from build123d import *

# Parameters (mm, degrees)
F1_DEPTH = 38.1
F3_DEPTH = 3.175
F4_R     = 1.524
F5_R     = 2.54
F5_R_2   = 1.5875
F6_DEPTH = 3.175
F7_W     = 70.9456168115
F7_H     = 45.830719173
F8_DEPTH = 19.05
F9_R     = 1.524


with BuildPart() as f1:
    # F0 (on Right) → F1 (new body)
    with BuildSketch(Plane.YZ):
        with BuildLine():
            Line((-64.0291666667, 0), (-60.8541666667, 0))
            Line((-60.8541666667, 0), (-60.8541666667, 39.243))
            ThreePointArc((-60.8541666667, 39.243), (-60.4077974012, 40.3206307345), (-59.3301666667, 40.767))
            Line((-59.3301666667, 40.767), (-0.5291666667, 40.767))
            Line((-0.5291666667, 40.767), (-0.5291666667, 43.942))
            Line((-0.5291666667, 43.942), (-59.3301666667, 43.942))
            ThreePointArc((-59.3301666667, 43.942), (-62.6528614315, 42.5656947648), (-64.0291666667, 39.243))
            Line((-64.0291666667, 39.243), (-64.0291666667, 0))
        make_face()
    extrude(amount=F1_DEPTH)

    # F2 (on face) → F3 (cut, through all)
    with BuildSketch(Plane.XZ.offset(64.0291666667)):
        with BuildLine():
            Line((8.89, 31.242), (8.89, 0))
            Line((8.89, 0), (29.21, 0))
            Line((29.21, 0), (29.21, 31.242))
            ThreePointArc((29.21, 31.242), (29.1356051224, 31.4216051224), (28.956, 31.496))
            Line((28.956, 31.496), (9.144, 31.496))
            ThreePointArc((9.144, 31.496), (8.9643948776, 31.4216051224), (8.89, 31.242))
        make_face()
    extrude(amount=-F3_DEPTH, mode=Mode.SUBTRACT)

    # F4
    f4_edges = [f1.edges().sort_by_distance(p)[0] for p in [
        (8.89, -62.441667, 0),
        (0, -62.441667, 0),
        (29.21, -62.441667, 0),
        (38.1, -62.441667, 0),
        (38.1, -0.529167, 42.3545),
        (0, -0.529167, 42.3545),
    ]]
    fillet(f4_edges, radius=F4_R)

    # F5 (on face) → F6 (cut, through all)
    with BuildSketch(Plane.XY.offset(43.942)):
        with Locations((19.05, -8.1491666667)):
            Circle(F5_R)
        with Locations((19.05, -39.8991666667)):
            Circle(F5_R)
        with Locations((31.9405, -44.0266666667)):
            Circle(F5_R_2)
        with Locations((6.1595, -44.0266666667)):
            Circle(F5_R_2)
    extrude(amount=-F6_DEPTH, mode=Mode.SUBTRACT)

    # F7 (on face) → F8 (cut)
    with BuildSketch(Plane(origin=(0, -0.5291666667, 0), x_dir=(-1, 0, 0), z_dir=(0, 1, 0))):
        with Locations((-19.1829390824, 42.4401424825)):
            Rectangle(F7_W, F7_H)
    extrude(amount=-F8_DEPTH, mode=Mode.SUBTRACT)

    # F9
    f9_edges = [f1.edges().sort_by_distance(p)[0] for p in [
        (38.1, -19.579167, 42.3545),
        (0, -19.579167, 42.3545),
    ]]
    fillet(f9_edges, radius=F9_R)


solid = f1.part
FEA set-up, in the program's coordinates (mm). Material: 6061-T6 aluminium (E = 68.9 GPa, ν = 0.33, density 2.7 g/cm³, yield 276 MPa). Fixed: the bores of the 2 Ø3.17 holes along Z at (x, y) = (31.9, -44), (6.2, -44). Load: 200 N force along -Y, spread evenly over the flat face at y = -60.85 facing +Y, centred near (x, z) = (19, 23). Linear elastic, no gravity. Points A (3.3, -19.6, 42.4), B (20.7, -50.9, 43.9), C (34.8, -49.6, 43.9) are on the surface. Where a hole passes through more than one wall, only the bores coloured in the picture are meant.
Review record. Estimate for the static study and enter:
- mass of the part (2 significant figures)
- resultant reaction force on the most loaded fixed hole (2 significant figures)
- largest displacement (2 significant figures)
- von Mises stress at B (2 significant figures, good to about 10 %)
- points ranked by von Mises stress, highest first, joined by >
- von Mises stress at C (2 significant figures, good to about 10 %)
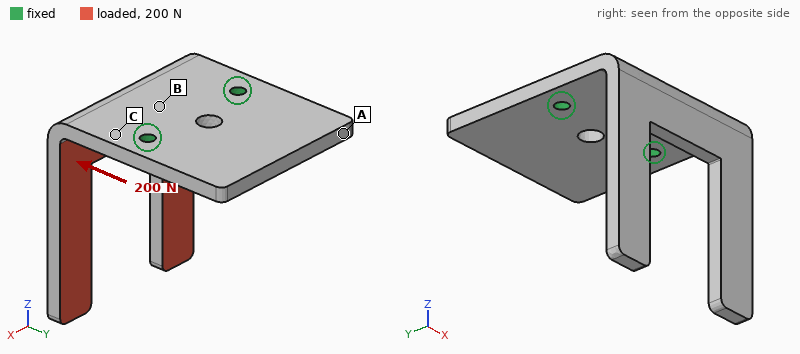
22 g
100 N
0.80 mm
47 MPa
C > B > A
64 MPa
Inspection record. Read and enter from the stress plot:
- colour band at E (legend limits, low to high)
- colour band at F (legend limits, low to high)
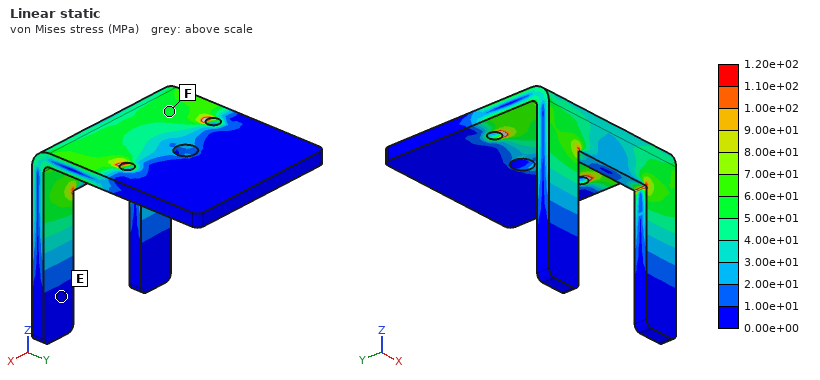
0.00e+00 to 1.00e+01 MPa
5.00e+01 to 6.00e+01 MPa
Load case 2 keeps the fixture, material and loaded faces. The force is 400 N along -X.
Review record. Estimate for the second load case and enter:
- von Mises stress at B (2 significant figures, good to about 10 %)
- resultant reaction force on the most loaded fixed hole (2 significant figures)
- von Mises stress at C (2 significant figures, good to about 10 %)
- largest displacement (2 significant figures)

38 MPa
420 N
69 MPa
0.40 mm
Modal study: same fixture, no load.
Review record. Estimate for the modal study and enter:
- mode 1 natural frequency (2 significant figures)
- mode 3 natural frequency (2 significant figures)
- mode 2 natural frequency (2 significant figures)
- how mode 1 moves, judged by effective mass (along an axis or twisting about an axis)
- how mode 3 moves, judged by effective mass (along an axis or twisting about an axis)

1100 Hz
2500 Hz
1500 Hz
along Y
along X
